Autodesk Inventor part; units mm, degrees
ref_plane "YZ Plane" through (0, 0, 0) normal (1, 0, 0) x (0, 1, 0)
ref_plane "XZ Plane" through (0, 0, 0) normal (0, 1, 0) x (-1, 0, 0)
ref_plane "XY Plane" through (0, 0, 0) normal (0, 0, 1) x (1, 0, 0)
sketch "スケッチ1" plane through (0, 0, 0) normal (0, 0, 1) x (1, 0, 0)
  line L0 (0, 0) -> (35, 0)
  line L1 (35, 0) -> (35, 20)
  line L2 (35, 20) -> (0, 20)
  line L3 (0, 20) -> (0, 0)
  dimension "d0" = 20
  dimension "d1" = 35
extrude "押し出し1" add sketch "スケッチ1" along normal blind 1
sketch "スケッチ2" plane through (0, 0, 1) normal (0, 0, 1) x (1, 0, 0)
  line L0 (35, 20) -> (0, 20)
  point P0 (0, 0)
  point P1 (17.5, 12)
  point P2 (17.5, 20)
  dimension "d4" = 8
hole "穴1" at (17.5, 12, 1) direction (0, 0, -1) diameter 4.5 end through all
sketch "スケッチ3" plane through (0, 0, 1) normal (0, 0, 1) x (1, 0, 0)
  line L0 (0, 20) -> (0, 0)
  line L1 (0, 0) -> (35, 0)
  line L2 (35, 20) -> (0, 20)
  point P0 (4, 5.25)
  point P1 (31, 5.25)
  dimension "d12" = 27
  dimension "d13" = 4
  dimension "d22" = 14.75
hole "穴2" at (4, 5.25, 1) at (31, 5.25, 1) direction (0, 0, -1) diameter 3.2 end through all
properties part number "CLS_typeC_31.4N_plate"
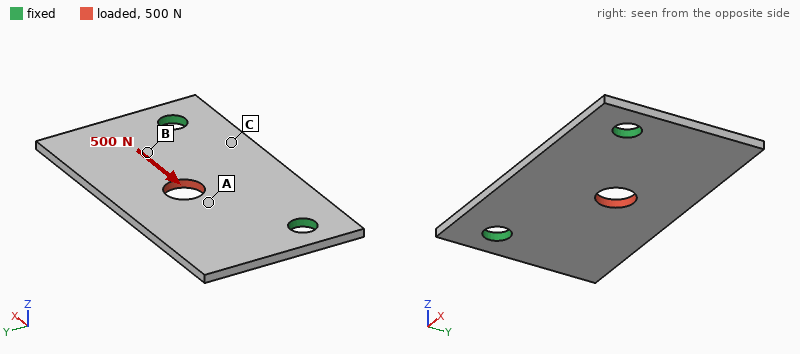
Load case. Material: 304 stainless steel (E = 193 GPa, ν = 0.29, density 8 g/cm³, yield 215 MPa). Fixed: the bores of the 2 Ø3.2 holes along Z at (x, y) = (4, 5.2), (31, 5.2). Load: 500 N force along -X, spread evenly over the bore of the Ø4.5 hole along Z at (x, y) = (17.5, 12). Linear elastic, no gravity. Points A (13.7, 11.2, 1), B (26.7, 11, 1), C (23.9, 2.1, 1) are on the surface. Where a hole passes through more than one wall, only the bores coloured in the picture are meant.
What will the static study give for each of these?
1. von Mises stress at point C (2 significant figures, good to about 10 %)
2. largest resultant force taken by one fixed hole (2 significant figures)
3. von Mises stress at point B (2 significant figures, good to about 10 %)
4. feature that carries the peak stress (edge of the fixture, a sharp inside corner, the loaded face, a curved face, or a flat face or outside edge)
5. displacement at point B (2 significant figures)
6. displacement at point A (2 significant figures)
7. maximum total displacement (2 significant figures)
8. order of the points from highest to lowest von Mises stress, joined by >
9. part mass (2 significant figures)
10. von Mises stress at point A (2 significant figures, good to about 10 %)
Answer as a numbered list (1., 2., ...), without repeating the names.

1. 9.7 MPa
2. 270 N
3. 26 MPa
4. edge of the fixture
5. 1.4 µm
6. 2.1 µm
7. 3.1 µm
8. A > B > C
9. 5.3 g
10. 38 MPa
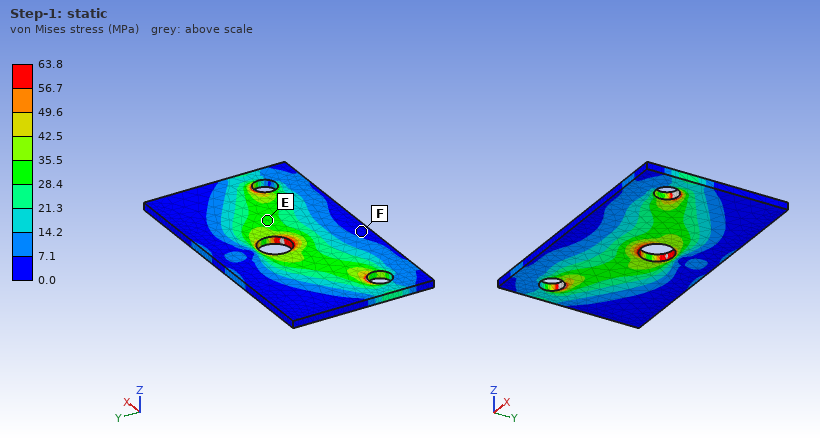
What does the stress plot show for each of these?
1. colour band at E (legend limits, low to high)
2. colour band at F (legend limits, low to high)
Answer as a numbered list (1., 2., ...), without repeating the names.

1. 28.4 to 35.5 MPa
2. 0.0 to 7.1 MPa
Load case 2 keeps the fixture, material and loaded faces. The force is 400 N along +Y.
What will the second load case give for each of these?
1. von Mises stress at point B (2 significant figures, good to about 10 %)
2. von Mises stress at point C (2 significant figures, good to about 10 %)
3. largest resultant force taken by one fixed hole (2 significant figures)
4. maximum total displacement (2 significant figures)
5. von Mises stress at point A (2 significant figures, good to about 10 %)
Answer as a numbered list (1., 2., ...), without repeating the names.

1. 23 MPa
2. 14 MPa
3. 220 N
4. 3.2 µm
5. 26 MPa
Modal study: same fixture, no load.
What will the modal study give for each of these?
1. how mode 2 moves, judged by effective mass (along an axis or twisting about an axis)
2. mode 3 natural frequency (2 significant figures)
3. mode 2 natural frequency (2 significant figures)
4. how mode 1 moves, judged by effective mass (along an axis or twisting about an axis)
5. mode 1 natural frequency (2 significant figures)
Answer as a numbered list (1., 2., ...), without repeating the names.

1. twisting about Y
2. 7400 Hz
3. 5600 Hz
4. along Z
5. 3300 Hz
